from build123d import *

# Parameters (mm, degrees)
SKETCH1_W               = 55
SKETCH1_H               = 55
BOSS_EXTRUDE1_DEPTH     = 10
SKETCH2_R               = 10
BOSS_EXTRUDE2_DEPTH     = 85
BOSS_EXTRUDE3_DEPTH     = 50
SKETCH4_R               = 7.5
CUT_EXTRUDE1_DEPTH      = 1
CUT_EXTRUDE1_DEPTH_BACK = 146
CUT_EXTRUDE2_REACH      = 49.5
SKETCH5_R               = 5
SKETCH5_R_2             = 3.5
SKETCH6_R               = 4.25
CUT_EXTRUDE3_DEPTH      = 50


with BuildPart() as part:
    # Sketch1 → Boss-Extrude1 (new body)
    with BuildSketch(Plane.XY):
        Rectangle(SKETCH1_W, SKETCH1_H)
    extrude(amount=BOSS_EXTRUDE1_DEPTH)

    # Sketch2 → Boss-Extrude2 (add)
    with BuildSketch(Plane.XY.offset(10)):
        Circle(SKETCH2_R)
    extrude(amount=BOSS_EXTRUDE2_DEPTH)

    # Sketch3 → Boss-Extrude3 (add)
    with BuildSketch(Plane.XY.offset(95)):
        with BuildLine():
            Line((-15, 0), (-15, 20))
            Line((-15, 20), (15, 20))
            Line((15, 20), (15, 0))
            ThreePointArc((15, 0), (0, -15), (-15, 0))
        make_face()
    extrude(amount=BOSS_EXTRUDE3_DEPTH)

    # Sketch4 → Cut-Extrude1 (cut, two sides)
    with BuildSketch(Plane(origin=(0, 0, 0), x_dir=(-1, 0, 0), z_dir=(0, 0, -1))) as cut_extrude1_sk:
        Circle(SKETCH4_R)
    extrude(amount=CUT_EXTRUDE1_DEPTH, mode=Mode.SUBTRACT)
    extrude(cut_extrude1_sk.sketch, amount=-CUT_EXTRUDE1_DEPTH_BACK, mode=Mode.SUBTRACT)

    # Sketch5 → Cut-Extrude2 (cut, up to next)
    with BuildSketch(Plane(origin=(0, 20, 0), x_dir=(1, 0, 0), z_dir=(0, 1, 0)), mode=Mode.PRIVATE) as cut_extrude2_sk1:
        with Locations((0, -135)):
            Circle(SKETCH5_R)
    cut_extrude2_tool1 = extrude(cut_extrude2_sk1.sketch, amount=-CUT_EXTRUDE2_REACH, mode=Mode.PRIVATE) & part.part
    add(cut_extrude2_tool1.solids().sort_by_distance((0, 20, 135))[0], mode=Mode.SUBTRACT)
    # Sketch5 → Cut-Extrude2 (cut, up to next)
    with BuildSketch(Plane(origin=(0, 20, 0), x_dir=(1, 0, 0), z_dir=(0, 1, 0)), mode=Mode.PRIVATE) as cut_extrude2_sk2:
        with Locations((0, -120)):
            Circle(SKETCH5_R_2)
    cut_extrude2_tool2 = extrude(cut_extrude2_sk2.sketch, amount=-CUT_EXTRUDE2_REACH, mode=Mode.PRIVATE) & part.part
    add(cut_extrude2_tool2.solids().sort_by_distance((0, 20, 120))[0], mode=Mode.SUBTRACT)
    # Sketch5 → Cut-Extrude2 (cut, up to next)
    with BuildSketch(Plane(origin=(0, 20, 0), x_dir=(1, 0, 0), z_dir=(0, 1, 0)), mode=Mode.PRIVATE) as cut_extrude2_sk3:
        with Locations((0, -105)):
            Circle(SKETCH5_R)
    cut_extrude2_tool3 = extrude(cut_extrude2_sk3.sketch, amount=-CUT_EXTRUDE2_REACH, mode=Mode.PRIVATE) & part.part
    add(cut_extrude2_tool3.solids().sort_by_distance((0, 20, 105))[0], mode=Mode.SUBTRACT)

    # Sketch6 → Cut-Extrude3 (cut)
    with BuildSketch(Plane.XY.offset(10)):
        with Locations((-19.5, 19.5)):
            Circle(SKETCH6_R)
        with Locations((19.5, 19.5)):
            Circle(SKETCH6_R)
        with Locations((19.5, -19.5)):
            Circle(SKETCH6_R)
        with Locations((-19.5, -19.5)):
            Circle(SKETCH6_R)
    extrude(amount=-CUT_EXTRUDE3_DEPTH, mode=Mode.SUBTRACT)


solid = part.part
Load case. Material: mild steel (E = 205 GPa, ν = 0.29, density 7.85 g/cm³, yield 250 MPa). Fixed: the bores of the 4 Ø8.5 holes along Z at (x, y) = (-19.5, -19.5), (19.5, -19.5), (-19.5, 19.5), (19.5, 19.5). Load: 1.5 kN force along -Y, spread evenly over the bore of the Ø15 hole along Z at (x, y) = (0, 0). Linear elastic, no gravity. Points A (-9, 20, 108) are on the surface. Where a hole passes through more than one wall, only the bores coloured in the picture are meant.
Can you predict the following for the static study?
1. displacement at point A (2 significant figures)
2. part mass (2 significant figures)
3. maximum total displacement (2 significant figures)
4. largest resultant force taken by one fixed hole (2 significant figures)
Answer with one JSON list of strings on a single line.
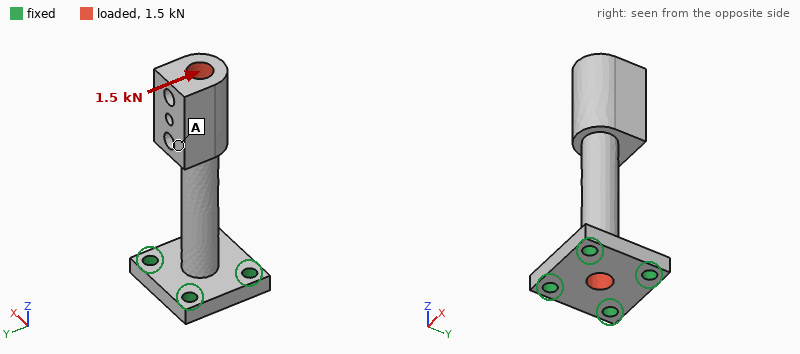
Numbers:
["0.34 mm", "580 g", "0.49 mm", "1.7 kN"]
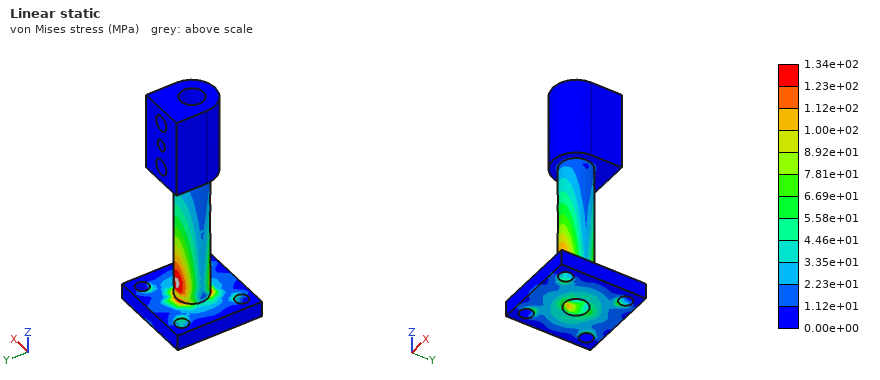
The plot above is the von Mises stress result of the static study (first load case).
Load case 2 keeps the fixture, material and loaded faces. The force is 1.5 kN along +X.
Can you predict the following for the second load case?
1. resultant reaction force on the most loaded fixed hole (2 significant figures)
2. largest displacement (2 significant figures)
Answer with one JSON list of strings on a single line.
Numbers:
["1.7 kN", "0.49 mm"]
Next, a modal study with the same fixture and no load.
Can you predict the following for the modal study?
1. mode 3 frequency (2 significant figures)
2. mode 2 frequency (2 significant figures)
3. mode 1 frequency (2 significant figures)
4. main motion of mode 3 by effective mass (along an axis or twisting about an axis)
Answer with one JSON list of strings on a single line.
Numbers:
["2100 Hz", "400 Hz", "400 Hz", "twisting about Z"]
